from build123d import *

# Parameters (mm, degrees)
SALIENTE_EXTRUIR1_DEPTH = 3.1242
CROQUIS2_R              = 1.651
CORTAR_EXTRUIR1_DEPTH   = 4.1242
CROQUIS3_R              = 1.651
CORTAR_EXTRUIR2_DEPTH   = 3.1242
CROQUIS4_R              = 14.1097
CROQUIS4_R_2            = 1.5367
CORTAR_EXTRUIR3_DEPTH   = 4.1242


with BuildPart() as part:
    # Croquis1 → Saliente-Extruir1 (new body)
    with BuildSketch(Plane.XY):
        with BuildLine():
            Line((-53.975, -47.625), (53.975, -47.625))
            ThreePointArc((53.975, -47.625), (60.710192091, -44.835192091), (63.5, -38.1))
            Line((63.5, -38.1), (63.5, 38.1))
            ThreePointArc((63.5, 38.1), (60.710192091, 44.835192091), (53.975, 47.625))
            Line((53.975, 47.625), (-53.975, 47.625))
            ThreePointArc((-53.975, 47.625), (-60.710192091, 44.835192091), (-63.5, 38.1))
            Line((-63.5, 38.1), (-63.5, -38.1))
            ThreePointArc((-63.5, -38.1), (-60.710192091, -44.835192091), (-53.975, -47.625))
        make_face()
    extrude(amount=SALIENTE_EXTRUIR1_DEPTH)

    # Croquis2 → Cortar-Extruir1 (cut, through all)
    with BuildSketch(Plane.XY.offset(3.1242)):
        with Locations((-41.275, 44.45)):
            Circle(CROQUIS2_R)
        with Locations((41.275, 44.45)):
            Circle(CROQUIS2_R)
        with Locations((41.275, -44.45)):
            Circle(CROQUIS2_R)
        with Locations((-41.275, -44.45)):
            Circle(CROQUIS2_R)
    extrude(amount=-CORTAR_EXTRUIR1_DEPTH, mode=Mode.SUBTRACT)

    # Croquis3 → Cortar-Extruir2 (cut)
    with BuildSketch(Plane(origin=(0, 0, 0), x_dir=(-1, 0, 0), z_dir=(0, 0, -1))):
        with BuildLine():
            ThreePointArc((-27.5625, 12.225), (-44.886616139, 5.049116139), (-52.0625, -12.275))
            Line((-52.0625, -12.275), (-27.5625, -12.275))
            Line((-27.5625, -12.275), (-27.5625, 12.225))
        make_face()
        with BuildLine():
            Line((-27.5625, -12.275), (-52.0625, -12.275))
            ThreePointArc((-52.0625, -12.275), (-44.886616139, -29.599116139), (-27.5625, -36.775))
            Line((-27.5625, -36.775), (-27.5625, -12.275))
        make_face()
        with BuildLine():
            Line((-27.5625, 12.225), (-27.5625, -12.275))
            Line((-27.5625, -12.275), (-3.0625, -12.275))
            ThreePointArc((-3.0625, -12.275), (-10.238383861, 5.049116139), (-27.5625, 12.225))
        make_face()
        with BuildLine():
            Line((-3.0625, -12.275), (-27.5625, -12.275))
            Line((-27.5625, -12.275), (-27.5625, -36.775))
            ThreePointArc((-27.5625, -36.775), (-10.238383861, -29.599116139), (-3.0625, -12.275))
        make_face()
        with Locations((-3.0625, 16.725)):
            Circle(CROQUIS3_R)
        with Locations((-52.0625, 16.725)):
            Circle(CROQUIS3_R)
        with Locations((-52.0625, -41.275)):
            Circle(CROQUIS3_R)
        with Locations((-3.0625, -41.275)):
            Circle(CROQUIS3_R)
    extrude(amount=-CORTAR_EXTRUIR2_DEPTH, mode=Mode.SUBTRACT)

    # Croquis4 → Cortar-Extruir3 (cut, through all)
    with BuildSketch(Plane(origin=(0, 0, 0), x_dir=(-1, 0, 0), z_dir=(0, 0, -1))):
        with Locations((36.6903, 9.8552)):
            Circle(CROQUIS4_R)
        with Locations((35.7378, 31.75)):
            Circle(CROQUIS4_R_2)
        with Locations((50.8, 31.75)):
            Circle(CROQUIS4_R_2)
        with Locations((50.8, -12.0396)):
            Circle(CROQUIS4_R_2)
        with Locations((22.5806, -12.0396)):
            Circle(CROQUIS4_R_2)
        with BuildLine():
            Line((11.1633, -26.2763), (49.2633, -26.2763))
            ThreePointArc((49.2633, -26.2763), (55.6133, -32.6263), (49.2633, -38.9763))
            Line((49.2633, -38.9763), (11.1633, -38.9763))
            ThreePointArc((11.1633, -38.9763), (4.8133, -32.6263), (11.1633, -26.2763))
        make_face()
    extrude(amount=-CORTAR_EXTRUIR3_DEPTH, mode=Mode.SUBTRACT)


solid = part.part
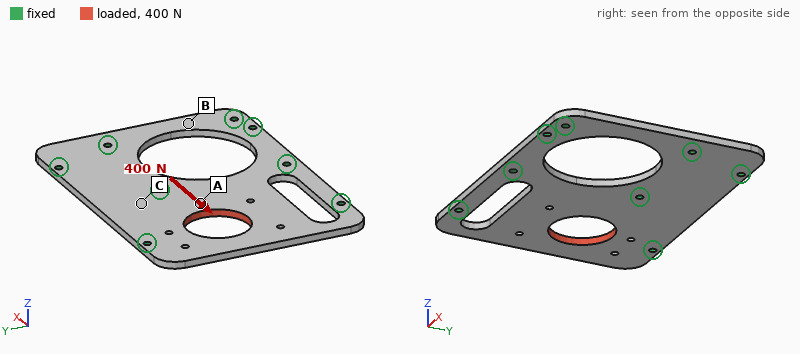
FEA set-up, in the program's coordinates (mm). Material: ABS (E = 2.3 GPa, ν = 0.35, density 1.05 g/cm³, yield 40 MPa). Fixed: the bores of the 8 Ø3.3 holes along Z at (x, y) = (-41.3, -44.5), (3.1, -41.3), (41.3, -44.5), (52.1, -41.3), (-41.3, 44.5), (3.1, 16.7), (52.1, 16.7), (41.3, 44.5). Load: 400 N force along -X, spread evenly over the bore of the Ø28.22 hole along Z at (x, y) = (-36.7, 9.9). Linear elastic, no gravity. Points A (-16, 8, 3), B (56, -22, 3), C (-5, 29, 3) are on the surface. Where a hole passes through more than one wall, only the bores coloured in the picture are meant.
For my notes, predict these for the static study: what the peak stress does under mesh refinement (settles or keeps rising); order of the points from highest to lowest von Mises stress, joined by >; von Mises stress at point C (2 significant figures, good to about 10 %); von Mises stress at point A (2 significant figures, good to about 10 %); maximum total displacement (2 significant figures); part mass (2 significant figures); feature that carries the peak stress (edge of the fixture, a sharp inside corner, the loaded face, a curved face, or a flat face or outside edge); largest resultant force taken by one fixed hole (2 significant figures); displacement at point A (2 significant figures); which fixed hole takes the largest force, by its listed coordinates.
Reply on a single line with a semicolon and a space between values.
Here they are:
keeps rising; A > C > B; 1.1 MPa; 2.2 MPa; 0.11 mm; 29 g; edge of the fixture; 180 N; 0.033 mm; (3.1, 16.7)
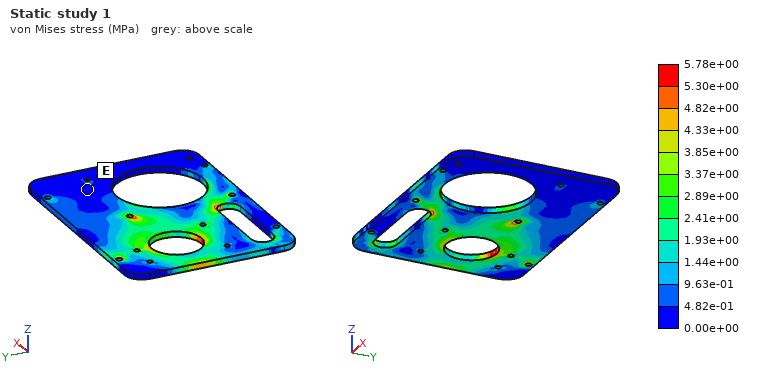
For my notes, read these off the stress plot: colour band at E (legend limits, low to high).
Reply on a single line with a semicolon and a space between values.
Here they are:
0.00e+00 to 4.82e-01 MPa
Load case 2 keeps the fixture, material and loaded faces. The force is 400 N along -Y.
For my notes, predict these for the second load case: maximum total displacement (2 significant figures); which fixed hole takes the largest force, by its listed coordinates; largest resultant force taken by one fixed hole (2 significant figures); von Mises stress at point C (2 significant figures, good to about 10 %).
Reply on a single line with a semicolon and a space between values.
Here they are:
90 µm; (-41.3, 44.5); 210 N; 1.3 MPa
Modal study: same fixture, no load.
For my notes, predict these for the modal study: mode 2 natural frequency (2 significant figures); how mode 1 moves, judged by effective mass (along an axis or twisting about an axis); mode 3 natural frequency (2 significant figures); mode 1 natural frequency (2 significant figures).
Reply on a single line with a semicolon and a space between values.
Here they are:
860 Hz; along Z; 1100 Hz; 440 Hz
